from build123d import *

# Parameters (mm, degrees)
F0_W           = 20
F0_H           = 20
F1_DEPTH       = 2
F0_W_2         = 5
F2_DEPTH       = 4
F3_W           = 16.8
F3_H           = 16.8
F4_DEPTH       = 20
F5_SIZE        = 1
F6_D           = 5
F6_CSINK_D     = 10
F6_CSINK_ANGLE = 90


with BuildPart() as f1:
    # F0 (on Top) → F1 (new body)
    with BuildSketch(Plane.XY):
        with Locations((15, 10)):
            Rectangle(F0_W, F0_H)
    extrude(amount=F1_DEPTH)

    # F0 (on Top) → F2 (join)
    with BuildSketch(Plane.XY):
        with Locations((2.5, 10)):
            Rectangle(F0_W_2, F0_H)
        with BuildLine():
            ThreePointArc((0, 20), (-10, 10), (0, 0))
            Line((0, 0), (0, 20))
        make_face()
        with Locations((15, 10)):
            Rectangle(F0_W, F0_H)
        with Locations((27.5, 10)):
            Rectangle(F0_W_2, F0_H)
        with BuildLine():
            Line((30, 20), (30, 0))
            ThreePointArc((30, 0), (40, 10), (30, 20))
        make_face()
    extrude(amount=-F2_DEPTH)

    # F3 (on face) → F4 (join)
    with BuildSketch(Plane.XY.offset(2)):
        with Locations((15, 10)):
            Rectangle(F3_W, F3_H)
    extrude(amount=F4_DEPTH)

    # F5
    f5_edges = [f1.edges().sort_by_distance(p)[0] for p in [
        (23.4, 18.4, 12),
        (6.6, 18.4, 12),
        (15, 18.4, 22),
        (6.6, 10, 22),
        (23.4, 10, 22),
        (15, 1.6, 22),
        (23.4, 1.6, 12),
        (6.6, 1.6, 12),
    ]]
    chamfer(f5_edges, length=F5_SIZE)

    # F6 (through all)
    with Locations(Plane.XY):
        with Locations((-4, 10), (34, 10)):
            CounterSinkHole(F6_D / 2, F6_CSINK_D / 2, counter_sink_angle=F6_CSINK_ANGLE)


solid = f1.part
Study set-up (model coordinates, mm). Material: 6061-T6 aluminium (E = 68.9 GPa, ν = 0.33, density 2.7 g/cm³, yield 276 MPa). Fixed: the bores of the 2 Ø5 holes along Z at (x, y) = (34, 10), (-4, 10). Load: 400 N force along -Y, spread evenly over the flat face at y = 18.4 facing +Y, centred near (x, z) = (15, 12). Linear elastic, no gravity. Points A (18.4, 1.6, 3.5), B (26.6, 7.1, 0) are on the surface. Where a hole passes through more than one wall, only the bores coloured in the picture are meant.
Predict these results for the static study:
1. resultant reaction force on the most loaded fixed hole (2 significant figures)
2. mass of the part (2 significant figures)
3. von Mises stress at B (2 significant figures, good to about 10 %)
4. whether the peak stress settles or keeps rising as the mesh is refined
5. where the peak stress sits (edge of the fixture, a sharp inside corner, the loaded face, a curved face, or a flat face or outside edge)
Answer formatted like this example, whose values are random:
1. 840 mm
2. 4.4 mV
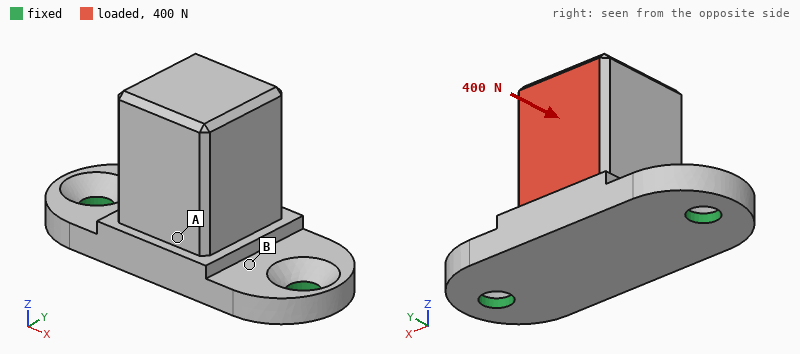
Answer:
1. 200 N
2. 26 g
3. 44 MPa
4. keeps rising
5. edge of the fixture
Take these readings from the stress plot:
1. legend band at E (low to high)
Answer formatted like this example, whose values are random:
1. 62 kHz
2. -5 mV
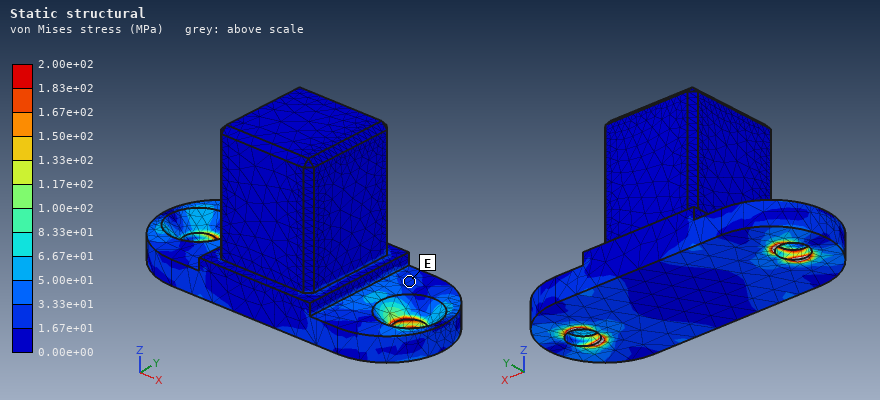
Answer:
1. 1.67e+01 to 3.33e+01 MPa
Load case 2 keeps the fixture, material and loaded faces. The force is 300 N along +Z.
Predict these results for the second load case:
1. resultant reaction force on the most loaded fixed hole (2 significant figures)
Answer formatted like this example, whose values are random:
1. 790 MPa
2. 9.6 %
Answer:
1. 230 N
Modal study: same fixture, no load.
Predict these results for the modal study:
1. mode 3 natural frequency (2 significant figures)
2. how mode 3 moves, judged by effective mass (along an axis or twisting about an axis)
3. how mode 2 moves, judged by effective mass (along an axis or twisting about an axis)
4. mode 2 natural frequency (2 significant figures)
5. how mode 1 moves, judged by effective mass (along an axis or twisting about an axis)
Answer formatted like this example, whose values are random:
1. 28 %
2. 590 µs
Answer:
1. 8800 Hz
2. along X
3. along Z
4. 8300 Hz
5. along Y
